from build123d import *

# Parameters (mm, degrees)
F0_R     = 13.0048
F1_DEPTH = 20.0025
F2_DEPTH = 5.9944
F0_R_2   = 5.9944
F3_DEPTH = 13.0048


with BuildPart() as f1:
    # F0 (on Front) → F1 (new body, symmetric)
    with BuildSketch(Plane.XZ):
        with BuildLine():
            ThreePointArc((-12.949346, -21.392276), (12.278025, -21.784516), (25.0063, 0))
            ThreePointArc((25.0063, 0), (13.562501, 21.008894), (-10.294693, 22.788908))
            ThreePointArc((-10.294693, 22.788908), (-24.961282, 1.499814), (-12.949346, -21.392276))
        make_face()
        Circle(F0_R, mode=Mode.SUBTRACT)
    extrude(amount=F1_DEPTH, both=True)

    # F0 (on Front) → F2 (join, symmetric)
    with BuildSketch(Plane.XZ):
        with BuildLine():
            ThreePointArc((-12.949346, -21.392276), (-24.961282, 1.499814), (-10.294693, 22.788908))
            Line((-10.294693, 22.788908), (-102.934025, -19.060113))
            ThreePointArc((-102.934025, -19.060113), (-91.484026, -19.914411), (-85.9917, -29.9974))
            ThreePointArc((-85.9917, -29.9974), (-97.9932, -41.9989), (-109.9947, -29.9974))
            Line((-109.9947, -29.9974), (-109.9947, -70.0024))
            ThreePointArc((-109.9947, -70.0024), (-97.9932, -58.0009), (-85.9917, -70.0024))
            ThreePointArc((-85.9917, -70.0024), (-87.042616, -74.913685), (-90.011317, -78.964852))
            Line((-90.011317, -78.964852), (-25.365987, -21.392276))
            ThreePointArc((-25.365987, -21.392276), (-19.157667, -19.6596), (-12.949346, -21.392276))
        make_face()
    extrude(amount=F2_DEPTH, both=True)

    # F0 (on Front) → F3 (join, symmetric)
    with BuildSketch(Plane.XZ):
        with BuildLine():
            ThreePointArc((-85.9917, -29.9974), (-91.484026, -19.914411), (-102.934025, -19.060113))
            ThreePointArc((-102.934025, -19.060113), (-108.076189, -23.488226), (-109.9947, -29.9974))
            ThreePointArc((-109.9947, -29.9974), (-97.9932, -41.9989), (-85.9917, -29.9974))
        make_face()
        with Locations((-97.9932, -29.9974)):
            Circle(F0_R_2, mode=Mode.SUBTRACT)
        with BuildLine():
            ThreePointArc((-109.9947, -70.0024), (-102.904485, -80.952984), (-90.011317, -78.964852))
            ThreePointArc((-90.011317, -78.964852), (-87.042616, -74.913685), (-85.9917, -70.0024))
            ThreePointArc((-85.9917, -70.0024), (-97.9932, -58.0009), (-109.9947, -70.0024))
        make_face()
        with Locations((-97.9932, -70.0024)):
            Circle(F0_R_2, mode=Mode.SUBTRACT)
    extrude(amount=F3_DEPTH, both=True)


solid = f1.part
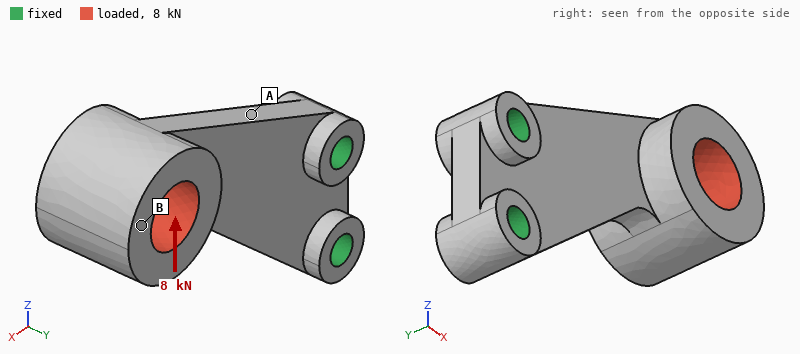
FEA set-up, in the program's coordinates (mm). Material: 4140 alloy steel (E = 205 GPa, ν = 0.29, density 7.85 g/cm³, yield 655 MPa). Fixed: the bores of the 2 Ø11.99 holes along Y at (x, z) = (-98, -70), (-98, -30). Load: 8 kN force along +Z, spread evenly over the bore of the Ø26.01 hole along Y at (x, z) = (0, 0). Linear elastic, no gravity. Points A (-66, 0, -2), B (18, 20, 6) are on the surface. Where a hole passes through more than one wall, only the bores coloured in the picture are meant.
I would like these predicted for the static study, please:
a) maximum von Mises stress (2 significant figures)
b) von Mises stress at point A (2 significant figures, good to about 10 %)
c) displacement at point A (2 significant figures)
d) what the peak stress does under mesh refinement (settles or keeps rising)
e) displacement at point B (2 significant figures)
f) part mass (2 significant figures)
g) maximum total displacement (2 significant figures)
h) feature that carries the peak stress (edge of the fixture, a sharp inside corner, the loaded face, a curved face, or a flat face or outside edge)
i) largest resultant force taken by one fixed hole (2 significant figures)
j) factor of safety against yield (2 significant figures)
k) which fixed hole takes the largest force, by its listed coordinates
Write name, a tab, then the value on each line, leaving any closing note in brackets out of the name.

maximum von Mises stress	190 MPa
von Mises stress at point A	120 MPa
displacement at point A	0.038 mm
what the peak stress does under mesh refinement	settles
displacement at point B	0.21 mm
part mass	940 g
maximum total displacement	0.23 mm
feature that carries the peak stress	a curved face
largest resultant force taken by one fixed hole	19 kN
factor of safety against yield	3.5
which fixed hole takes the largest force, by its listed coordinates	(-98, -70)
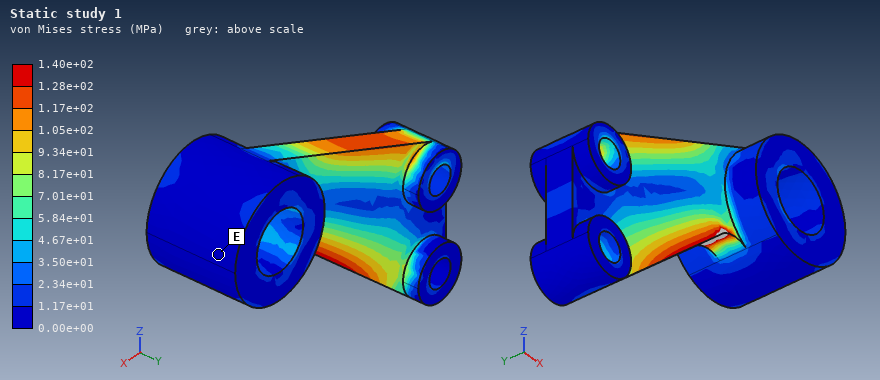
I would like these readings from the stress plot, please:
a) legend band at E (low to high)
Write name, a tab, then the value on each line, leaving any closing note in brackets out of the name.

legend band at E	0.00e+00 to 1.17e+01 MPa
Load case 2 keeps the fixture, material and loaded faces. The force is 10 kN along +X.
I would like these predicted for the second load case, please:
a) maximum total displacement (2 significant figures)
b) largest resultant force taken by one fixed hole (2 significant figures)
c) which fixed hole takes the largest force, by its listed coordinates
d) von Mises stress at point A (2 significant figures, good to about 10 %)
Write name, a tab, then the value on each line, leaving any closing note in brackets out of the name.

maximum total displacement	99 µm
largest resultant force taken by one fixed hole	16 kN
which fixed hole takes the largest force, by its listed coordinates	(-98, -30)
von Mises stress at point A	76 MPa
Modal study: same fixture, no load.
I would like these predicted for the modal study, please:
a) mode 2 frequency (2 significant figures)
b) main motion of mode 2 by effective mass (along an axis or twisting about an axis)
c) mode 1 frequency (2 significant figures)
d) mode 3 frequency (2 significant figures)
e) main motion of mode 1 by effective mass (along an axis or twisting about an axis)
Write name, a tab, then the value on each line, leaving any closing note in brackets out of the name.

mode 2 frequency	1500 Hz
main motion of mode 2 by effective mass	along Z
mode 1 frequency	460 Hz
mode 3 frequency	1900 Hz
main motion of mode 1 by effective mass	along Y
